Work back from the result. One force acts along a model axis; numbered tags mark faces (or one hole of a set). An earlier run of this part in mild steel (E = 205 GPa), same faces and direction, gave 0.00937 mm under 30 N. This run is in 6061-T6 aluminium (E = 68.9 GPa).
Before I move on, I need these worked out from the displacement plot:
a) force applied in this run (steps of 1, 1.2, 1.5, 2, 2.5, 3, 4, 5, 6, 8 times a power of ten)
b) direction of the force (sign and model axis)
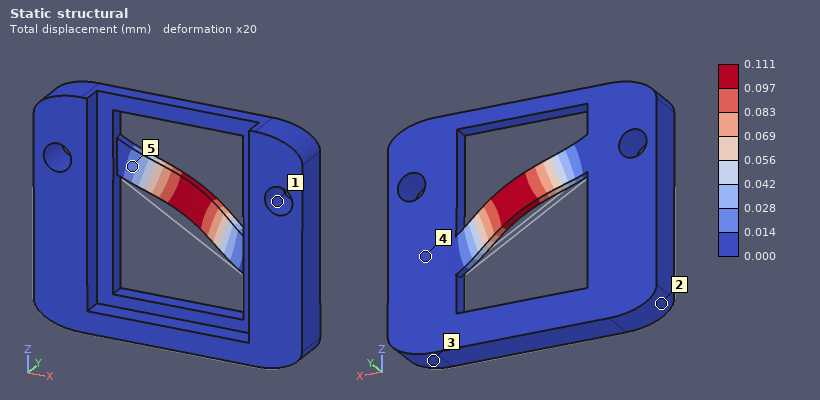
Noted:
120 N
+Y
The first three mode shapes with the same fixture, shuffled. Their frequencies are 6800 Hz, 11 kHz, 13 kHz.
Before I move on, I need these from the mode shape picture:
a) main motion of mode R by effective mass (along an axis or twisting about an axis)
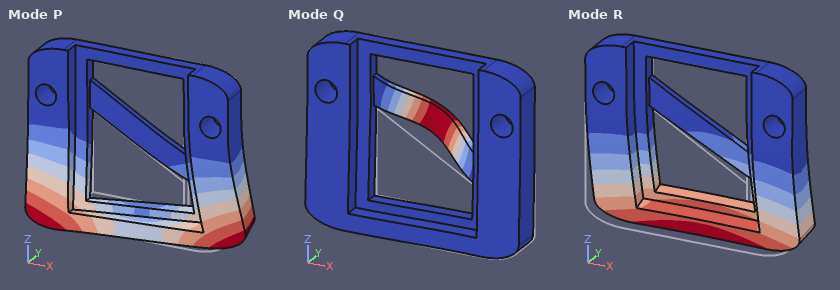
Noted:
along Y
